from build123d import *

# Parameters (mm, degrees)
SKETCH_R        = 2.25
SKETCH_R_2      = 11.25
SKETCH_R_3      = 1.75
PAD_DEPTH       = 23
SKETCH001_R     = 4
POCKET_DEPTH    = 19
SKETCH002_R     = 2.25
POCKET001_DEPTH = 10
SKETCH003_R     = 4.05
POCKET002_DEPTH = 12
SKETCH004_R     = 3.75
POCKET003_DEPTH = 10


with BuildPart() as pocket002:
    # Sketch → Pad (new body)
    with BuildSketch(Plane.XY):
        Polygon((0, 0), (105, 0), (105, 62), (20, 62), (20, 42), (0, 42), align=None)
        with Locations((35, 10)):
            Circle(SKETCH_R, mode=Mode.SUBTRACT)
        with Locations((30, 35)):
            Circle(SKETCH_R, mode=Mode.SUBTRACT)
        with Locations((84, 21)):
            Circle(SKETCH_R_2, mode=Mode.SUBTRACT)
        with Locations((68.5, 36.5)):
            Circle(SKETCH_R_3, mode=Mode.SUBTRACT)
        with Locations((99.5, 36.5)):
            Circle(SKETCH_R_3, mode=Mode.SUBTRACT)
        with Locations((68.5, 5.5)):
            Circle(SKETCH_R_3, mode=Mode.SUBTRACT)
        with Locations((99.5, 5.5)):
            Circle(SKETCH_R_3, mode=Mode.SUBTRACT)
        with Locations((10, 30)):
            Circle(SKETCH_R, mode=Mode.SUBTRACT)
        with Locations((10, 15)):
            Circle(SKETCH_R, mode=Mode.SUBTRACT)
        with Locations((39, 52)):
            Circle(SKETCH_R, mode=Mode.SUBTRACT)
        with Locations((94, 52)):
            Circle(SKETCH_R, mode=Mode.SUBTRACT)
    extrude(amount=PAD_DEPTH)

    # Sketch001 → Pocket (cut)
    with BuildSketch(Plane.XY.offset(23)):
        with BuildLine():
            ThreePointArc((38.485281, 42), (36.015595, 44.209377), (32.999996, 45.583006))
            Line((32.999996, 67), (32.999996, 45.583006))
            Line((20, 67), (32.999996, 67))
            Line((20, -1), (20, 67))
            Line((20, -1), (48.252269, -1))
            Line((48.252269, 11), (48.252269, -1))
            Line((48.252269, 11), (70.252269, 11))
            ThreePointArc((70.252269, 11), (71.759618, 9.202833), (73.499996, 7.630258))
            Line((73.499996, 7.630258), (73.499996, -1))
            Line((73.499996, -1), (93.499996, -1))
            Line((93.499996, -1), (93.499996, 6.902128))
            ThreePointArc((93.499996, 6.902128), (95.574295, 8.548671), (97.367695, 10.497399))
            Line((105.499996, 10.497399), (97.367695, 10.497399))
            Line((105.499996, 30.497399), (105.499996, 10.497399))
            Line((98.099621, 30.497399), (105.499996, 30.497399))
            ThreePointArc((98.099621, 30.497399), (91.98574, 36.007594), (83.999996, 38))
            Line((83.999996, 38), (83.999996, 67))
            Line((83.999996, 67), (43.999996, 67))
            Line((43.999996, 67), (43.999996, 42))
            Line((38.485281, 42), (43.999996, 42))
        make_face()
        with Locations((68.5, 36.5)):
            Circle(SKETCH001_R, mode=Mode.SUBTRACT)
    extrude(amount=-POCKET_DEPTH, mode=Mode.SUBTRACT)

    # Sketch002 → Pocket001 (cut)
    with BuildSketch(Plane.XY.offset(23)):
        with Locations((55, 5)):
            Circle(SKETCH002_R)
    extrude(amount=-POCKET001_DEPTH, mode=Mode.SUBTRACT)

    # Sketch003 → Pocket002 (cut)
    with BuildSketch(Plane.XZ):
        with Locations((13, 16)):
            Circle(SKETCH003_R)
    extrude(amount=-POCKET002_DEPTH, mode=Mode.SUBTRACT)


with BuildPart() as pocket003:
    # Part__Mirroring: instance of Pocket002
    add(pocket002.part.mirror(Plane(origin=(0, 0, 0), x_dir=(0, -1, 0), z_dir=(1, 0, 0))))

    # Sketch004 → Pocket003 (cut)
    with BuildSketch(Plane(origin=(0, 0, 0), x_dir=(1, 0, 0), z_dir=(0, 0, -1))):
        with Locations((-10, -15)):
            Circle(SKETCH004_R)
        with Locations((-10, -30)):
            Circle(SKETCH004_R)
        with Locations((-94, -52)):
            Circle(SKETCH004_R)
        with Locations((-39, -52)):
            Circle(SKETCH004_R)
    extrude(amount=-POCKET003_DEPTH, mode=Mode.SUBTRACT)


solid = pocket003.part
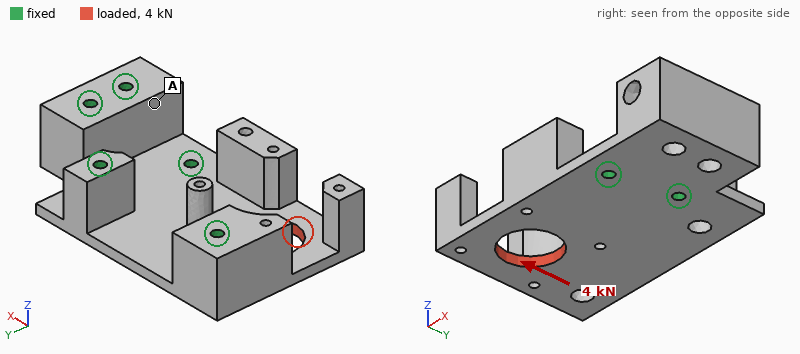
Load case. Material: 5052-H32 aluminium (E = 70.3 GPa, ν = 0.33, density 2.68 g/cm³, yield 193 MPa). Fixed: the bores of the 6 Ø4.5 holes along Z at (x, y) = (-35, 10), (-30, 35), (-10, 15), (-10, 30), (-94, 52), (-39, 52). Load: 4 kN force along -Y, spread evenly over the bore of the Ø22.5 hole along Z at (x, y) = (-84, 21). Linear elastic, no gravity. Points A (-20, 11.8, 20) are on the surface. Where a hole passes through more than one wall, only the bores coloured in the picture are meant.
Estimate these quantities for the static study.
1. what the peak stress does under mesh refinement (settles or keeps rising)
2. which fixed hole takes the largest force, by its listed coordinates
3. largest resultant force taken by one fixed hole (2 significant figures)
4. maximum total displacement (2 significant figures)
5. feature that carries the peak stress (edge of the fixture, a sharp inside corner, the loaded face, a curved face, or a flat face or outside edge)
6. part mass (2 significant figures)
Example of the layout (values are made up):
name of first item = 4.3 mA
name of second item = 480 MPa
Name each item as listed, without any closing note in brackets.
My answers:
what the peak stress does under mesh refinement = keeps rising
which fixed hole takes the largest force, by its listed coordinates = (-94, 52)
largest resultant force taken by one fixed hole = 2.6 kN
maximum total displacement = 50 µm
feature that carries the peak stress = edge of the fixture
part mass = 150 g
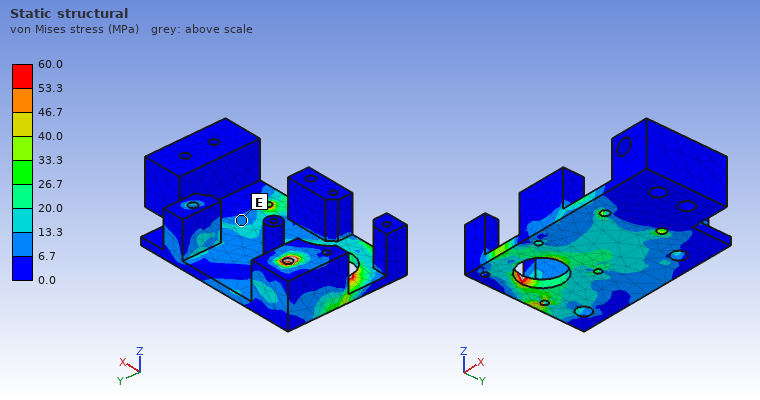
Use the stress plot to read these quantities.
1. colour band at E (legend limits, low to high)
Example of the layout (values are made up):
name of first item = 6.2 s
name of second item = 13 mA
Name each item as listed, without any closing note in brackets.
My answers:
colour band at E = 6.7 to 13.3 MPa
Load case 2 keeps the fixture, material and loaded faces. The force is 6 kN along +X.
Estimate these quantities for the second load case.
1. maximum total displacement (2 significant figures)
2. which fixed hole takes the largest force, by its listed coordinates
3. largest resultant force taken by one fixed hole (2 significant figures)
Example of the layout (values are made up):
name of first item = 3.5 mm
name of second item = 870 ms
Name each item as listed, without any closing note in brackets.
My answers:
maximum total displacement = 41 µm
which fixed hole takes the largest force, by its listed coordinates = (-35, 10)
largest resultant force taken by one fixed hole = 2.4 kN
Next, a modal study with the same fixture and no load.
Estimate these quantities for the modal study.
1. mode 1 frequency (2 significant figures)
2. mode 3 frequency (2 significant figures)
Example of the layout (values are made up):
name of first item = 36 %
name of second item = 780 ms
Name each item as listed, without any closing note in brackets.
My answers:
mode 1 frequency = 1600 Hz
mode 3 frequency = 4400 Hz
